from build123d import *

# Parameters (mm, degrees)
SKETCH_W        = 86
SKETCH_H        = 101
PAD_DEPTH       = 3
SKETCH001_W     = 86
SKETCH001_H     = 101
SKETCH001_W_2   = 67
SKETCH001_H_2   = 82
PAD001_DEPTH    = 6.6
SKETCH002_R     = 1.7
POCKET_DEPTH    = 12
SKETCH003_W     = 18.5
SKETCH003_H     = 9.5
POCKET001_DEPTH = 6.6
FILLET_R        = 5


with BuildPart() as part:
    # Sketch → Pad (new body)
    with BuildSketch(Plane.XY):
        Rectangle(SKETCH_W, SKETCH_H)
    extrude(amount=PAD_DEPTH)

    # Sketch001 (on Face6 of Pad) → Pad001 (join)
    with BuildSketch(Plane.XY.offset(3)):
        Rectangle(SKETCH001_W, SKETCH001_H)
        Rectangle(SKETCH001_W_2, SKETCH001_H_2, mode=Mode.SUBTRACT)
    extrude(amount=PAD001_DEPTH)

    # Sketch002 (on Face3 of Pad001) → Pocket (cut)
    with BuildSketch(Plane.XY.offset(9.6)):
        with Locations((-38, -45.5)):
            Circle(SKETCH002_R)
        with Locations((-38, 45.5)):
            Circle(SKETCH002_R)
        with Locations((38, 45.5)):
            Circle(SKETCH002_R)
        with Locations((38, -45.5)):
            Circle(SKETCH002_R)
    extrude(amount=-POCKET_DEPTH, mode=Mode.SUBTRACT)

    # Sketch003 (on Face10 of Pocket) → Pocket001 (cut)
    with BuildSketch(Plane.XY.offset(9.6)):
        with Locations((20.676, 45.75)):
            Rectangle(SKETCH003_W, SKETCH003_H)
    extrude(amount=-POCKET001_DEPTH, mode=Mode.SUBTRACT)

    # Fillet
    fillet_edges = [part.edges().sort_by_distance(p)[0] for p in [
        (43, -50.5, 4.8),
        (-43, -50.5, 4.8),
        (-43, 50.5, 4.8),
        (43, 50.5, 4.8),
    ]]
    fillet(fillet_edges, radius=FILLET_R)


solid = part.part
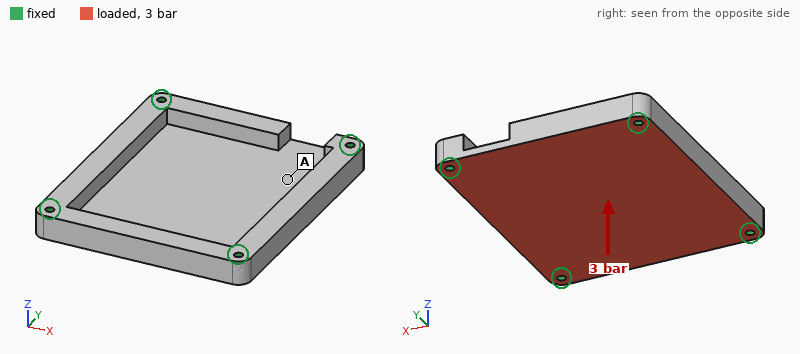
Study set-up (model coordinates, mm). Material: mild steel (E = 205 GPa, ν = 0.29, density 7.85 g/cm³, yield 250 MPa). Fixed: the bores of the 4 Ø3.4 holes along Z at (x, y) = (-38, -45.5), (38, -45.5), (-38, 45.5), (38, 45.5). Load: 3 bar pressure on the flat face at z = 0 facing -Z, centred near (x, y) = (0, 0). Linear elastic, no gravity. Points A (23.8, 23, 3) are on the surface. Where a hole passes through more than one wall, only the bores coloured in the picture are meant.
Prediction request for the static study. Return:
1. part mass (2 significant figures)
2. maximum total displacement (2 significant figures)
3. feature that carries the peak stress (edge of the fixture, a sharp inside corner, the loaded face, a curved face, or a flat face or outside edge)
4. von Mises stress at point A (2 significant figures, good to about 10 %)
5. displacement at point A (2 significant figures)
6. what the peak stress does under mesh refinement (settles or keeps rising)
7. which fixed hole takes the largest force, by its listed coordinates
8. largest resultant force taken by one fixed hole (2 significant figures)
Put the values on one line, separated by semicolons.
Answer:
360 g; 50 µm; edge of the fixture; 12 MPa; 20 µm; keeps rising; (-38, 45.5); 940 N
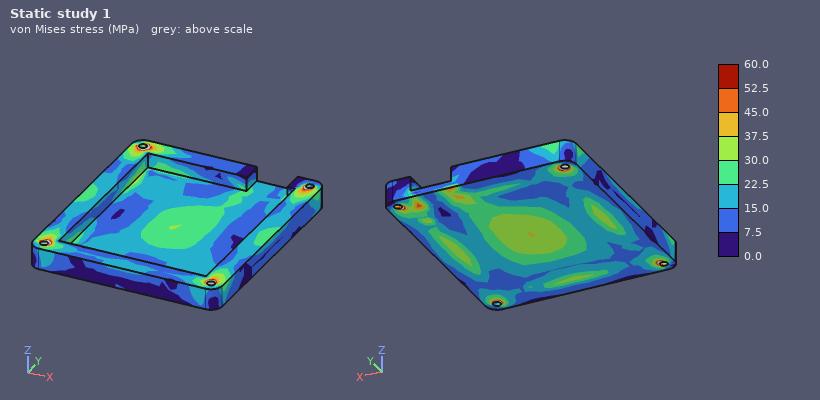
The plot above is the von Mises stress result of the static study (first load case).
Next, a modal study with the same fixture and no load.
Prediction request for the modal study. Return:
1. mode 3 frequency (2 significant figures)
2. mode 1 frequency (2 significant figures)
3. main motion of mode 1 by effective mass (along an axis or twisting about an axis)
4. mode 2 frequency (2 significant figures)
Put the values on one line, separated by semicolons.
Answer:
5200 Hz; 3200 Hz; along Z; 5000 Hz
